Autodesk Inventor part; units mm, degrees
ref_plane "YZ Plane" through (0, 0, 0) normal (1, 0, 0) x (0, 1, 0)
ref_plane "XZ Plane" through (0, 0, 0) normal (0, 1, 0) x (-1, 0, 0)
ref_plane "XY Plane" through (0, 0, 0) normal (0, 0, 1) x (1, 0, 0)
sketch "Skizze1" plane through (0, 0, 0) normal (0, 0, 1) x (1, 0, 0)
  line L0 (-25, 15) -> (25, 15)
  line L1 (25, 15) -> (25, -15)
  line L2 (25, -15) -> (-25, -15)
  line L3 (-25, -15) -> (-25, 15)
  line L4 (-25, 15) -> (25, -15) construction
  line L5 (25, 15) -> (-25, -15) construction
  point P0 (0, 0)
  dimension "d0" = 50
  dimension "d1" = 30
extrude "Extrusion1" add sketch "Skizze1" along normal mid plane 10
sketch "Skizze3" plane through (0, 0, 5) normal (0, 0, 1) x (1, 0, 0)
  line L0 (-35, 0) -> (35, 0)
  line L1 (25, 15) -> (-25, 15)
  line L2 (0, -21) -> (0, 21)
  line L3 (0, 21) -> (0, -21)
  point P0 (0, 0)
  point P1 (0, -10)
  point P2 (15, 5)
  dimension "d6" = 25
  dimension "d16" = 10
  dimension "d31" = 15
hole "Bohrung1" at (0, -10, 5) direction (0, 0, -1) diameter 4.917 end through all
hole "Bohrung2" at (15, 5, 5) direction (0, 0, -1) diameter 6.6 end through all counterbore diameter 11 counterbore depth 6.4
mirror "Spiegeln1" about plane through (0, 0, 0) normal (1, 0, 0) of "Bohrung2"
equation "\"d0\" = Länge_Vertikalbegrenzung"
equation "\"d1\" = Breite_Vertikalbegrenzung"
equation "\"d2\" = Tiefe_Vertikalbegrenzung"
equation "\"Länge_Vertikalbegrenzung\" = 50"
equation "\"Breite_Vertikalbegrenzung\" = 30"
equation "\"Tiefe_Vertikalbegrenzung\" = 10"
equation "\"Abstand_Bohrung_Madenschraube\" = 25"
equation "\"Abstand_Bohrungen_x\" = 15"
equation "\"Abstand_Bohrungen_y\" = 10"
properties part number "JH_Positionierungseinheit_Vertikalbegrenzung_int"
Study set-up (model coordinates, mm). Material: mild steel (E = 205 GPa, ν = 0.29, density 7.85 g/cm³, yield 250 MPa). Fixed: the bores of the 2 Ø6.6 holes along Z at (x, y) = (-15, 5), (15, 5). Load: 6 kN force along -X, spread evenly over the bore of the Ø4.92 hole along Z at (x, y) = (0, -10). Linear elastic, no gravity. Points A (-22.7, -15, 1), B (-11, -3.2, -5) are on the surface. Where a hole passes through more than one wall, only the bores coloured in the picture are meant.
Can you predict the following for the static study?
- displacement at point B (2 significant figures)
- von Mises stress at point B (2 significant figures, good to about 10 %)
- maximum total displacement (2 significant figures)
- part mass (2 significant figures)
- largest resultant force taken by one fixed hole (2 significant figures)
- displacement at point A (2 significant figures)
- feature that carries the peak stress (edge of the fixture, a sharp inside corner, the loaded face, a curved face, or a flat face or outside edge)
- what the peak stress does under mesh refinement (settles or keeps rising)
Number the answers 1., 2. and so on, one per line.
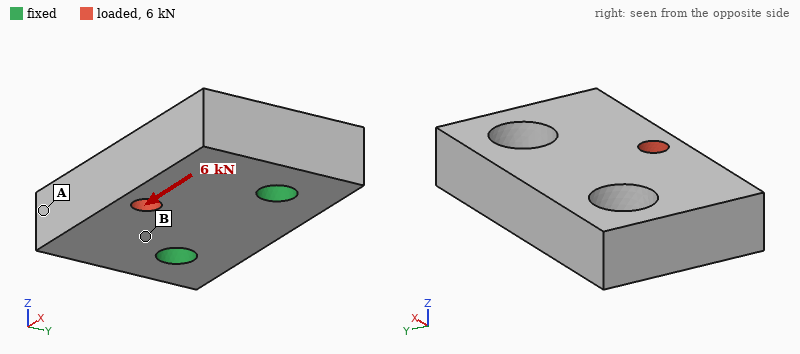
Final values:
1. 2.8 µm
2. 48 MPa
3. 7.1 µm
4. 100 g
5. 4.0 kN
6. 6.4 µm
7. edge of the fixture
8. keeps rising
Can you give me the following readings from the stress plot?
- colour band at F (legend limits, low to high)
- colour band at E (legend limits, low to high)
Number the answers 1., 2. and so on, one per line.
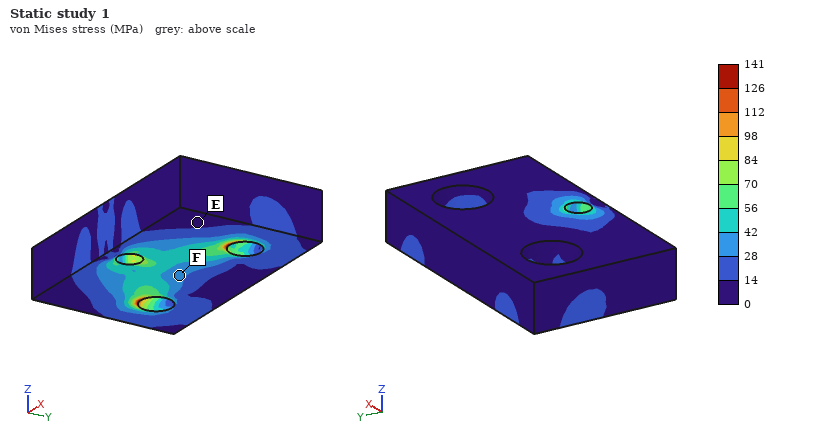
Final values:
1. 28 to 42 MPa
2. 0 to 14 MPa
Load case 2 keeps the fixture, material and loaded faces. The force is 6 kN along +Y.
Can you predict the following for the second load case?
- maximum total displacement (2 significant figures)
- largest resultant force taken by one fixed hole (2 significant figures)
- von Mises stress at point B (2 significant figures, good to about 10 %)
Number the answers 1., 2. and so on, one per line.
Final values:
1. 17 µm
2. 3.1 kN
3. 43 MPa
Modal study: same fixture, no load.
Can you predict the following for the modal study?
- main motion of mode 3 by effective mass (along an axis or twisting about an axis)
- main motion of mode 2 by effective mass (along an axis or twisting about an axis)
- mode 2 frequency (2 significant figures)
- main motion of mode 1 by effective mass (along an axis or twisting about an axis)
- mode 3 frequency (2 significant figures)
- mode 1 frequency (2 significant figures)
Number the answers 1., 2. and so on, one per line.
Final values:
1. along X
2. twisting about Y
3. 15 kHz
4. along Z
5. 22 kHz
6. 8100 Hz
